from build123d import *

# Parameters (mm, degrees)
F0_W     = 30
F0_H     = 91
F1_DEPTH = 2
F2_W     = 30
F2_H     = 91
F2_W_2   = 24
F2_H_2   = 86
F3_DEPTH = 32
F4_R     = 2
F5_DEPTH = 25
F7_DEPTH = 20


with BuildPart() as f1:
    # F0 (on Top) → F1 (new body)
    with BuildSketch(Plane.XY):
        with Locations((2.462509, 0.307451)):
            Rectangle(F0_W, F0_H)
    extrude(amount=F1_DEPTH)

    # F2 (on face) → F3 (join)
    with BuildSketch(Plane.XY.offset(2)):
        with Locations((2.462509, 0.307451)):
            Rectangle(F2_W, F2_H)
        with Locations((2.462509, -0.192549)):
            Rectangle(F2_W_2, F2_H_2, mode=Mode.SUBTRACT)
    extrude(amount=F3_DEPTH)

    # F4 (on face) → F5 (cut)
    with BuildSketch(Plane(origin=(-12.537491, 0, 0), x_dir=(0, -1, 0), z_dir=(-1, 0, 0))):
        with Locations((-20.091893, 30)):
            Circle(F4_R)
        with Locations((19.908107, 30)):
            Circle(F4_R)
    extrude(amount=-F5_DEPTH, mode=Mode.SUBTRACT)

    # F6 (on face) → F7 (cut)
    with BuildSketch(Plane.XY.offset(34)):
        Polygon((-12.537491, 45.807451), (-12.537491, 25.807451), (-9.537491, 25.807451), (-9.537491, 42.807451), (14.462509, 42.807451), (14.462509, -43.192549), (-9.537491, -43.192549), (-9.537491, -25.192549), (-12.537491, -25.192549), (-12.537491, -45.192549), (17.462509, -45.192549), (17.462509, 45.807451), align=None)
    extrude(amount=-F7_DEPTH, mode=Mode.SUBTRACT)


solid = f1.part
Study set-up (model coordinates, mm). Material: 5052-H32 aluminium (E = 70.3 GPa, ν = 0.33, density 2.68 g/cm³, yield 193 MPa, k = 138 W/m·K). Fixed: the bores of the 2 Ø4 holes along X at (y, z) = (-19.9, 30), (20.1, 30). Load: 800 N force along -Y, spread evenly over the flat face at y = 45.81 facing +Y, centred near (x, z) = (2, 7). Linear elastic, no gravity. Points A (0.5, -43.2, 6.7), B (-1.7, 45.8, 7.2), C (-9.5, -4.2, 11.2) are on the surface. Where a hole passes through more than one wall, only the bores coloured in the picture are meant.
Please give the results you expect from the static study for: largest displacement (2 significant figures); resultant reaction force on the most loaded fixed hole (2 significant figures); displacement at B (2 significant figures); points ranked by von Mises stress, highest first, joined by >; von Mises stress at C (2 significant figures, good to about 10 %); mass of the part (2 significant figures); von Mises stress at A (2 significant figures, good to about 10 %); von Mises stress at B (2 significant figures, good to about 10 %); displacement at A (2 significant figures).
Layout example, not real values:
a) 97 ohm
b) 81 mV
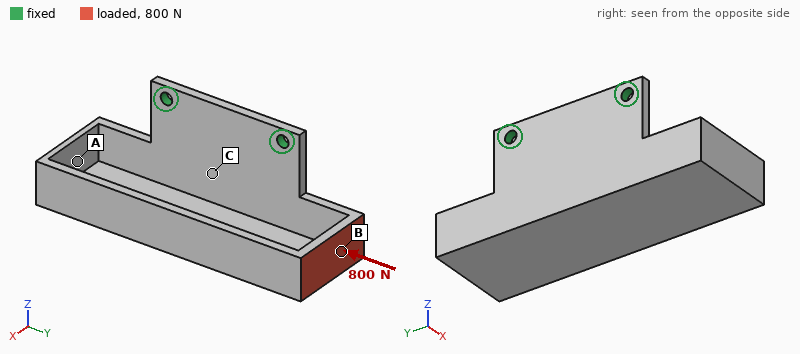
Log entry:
a) 0.65 mm
b) 650 N
c) 0.47 mm
d) C > B > A
e) 73 MPa
f) 44 g
g) 25 MPa
h) 50 MPa
i) 0.45 mm
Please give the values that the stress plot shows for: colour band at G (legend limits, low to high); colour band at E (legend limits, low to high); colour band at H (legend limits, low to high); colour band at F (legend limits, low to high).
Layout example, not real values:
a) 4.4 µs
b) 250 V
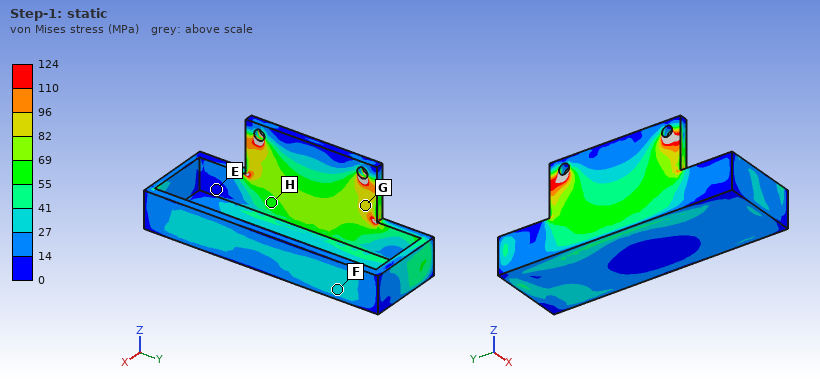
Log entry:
a) 82 to 96 MPa
b) 0 to 14 MPa
c) 55 to 69 MPa
d) 27 to 41 MPa
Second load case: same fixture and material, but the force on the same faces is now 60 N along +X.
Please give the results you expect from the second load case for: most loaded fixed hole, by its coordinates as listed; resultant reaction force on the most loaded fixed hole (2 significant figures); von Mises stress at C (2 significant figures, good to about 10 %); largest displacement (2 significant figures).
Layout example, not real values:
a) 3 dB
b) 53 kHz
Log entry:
a) (20.1, 30)
b) 95 N
c) 13 MPa
d) 0.19 mm
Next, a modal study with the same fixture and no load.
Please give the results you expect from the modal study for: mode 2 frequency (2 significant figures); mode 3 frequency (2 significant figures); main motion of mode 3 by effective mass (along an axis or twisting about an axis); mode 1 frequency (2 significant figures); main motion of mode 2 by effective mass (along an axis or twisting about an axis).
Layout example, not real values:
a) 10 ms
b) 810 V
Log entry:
a) 830 Hz
b) 1500 Hz
c) along X
d) 600 Hz
e) along Y
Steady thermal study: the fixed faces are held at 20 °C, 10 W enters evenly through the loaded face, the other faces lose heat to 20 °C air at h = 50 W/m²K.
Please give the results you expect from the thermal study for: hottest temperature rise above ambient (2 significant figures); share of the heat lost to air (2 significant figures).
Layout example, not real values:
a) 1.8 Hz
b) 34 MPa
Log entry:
a) 25 K
b) 54 %
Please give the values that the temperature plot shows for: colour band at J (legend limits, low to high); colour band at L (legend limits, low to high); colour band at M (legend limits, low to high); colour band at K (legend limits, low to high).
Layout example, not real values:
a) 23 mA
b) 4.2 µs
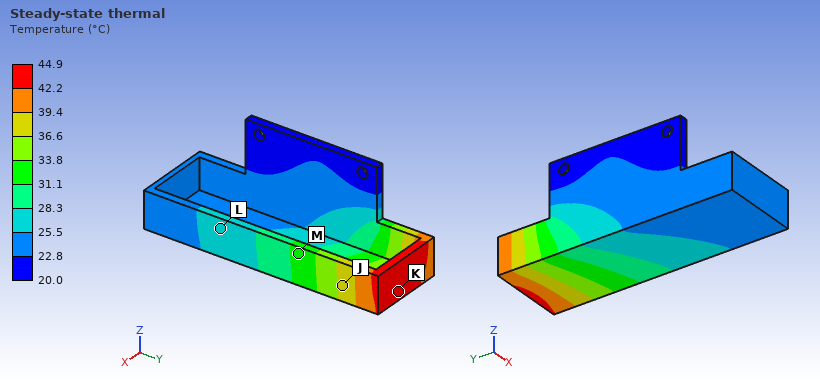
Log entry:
a) 36.6 to 39.4 °C
b) 25.5 to 28.3 °C
c) 31.1 to 33.8 °C
d) 42.2 to 44.9 °C
